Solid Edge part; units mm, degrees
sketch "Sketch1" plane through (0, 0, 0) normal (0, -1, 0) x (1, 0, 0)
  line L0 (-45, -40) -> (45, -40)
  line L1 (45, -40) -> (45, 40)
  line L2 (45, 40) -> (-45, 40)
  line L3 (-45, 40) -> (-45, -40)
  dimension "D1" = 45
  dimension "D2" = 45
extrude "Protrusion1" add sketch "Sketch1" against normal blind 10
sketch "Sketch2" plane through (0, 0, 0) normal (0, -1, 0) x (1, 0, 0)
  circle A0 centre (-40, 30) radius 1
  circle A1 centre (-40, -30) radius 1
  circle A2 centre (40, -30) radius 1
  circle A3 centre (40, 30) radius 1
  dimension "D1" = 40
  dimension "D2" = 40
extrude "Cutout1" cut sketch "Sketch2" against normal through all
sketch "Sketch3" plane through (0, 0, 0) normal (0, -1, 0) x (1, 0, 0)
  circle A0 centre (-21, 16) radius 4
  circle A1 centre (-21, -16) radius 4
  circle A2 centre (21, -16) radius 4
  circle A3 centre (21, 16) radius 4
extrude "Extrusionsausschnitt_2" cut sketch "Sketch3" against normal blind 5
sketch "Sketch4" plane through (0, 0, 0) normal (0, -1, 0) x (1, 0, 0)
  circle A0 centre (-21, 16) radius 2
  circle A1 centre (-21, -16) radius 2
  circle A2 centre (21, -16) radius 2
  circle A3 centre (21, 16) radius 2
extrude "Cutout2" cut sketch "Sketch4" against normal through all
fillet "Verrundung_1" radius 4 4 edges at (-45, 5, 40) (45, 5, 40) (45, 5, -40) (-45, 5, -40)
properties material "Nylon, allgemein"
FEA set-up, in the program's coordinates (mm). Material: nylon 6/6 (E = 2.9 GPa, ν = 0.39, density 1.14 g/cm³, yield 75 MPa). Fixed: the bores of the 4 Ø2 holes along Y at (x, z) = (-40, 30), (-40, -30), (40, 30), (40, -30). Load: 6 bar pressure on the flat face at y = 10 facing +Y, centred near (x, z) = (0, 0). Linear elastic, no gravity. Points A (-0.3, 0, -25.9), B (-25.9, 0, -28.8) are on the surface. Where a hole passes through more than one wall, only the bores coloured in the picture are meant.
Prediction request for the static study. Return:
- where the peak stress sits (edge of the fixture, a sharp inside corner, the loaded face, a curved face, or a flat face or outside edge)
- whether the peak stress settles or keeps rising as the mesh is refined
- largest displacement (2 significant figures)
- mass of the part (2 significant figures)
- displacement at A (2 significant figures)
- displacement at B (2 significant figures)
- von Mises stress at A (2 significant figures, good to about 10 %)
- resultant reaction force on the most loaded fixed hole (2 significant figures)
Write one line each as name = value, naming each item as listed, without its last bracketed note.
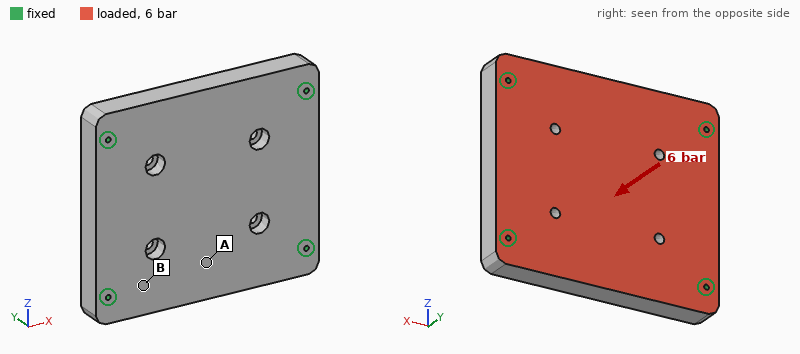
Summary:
where the peak stress sits = edge of the fixture
whether the peak stress settles or keeps rising as the mesh is refined = keeps rising
largest displacement = 0.70 mm
mass of the part = 80 g
displacement at A = 0.64 mm
displacement at B = 0.33 mm
von Mises stress at A = 14 MPa
resultant reaction force on the most loaded fixed hole = 1.1 kN
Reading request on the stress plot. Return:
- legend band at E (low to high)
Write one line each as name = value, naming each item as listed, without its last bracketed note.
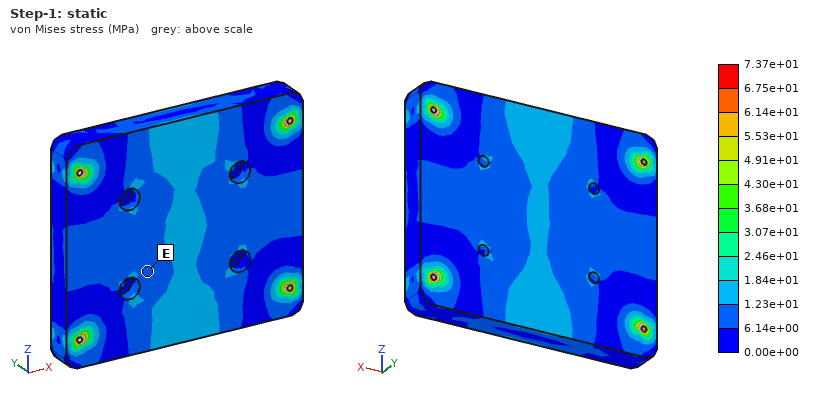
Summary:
legend band at E = 6.14e+00 to 1.23e+01 MPa
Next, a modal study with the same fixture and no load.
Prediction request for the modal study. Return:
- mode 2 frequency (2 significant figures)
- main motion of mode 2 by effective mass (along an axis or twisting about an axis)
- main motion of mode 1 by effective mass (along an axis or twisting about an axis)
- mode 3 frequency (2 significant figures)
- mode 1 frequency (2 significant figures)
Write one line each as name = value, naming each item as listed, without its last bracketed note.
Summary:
mode 2 frequency = 2300 Hz
main motion of mode 2 by effective mass = twisting about X
main motion of mode 1 by effective mass = along Y
mode 3 frequency = 3100 Hz
mode 1 frequency = 1600 Hz
